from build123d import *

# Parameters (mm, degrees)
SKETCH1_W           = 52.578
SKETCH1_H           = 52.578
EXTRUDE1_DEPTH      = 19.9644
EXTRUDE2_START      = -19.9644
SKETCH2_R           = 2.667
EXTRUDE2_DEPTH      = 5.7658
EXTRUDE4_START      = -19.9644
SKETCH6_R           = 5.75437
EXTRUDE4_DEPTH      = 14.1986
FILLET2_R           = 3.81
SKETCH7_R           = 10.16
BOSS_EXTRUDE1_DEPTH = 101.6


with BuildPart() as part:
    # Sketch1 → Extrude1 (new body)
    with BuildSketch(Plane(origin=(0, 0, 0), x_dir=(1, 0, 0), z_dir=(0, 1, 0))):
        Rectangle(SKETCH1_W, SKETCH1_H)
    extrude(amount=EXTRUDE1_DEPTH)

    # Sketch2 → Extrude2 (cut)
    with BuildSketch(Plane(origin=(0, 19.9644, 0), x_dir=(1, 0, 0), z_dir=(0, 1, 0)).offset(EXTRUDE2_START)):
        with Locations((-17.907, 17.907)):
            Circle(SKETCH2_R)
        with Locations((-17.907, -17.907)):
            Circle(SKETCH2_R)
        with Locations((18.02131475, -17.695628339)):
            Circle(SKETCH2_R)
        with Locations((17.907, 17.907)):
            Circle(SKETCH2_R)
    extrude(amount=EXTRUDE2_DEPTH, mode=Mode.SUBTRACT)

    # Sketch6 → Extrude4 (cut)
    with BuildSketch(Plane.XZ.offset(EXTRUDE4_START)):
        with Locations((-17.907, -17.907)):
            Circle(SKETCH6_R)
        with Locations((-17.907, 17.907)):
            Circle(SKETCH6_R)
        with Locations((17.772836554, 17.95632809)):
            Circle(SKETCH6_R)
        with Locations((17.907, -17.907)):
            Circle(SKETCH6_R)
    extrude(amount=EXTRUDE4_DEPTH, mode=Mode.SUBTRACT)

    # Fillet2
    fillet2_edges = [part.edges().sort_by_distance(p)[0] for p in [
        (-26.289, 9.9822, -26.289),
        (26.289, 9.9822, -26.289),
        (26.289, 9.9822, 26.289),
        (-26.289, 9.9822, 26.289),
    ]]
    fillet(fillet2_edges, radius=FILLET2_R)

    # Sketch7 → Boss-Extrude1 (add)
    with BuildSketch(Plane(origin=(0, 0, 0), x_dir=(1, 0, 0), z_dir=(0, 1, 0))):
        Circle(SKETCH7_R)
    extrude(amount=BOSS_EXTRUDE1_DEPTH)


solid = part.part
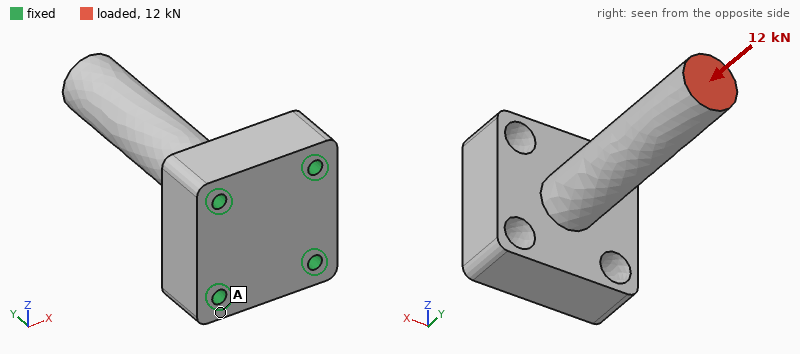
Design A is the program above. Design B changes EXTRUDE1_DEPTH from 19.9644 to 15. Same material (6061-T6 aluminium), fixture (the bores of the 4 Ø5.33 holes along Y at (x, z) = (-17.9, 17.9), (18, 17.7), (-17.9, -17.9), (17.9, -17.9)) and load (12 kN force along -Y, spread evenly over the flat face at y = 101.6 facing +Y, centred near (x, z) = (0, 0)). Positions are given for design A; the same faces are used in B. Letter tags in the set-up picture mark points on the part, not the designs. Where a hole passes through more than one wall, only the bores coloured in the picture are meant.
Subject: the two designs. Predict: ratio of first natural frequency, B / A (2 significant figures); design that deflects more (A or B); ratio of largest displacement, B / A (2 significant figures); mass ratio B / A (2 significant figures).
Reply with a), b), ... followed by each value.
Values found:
a) 0.89
b) B
c) 1.1
d) 0.87
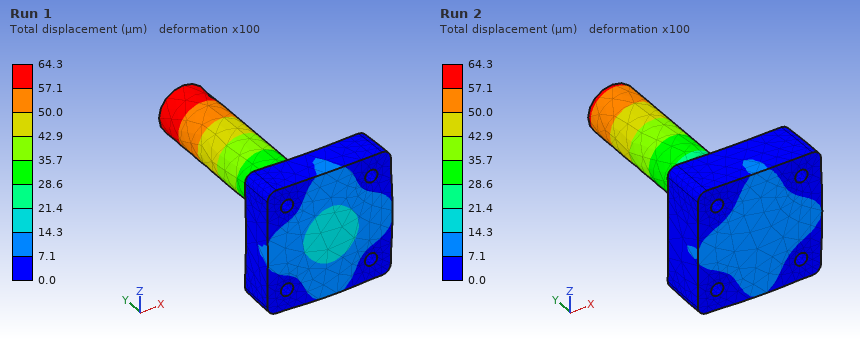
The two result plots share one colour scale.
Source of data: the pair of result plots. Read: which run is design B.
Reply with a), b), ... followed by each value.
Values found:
a) Run 1
